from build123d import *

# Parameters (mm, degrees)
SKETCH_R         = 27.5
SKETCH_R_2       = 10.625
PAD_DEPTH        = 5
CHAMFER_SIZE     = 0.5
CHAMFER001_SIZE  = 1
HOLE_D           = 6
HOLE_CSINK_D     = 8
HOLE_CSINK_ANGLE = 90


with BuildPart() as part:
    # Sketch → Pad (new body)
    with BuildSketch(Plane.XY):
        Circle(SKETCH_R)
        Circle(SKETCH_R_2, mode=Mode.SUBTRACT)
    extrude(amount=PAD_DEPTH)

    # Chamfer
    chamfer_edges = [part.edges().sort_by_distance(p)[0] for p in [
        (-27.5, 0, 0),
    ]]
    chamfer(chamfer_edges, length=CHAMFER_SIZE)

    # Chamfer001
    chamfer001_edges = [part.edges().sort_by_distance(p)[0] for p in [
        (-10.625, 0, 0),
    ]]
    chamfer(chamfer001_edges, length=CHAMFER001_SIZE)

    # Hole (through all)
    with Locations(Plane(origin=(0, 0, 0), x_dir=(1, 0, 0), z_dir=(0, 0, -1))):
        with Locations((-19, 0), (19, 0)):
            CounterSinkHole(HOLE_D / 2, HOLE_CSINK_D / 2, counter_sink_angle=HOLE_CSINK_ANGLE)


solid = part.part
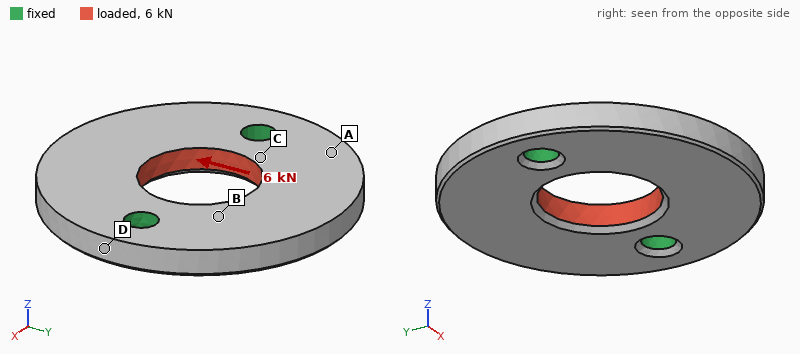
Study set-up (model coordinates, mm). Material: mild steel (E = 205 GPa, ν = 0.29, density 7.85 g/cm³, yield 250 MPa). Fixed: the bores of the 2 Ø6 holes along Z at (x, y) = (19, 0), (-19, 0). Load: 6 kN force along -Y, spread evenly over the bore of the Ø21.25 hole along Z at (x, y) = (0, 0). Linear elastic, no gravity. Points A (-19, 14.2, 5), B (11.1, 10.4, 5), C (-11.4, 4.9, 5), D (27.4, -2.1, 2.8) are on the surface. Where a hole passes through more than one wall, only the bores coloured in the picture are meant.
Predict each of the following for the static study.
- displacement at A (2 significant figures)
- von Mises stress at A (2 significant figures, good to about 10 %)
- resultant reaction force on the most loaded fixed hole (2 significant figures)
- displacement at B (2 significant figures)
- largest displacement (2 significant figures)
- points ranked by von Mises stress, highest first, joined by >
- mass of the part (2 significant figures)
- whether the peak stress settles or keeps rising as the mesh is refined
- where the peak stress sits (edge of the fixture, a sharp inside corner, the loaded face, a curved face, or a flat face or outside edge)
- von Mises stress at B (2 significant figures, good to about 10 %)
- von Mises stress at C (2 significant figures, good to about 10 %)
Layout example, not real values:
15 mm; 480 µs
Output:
1.6 µm; 15 MPa; 3.0 kN; 2.5 µm; 4.9 µm; C > B > A > D; 77 g; keeps rising; edge of the fixture; 27 MPa; 37 MPa
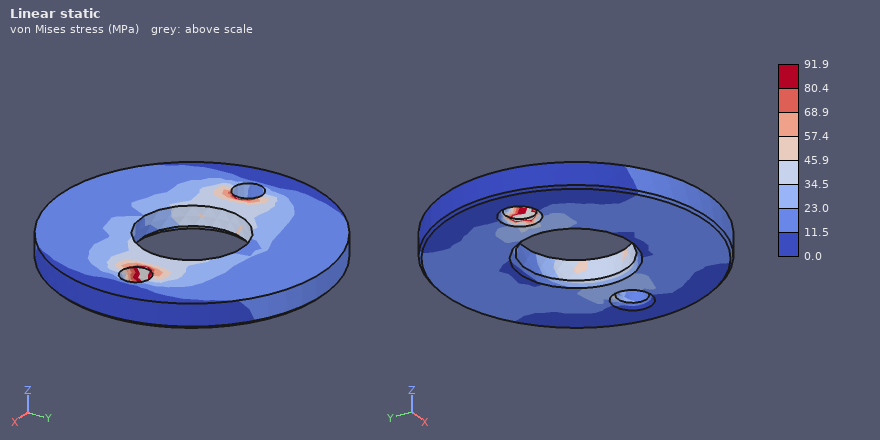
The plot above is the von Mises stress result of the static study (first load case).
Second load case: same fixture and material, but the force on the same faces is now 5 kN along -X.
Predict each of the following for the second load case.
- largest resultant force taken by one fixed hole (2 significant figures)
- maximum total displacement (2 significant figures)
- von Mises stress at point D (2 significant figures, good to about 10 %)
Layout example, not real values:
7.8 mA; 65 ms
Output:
2.5 kN; 3.1 µm; 21 MPa
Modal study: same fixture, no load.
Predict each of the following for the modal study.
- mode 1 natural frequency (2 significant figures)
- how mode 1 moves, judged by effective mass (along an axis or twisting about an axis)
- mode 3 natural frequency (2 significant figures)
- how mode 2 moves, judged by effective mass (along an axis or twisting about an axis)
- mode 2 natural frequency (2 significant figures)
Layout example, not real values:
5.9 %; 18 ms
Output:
5400 Hz; twisting about X; 13 kHz; along Z; 5700 Hz
